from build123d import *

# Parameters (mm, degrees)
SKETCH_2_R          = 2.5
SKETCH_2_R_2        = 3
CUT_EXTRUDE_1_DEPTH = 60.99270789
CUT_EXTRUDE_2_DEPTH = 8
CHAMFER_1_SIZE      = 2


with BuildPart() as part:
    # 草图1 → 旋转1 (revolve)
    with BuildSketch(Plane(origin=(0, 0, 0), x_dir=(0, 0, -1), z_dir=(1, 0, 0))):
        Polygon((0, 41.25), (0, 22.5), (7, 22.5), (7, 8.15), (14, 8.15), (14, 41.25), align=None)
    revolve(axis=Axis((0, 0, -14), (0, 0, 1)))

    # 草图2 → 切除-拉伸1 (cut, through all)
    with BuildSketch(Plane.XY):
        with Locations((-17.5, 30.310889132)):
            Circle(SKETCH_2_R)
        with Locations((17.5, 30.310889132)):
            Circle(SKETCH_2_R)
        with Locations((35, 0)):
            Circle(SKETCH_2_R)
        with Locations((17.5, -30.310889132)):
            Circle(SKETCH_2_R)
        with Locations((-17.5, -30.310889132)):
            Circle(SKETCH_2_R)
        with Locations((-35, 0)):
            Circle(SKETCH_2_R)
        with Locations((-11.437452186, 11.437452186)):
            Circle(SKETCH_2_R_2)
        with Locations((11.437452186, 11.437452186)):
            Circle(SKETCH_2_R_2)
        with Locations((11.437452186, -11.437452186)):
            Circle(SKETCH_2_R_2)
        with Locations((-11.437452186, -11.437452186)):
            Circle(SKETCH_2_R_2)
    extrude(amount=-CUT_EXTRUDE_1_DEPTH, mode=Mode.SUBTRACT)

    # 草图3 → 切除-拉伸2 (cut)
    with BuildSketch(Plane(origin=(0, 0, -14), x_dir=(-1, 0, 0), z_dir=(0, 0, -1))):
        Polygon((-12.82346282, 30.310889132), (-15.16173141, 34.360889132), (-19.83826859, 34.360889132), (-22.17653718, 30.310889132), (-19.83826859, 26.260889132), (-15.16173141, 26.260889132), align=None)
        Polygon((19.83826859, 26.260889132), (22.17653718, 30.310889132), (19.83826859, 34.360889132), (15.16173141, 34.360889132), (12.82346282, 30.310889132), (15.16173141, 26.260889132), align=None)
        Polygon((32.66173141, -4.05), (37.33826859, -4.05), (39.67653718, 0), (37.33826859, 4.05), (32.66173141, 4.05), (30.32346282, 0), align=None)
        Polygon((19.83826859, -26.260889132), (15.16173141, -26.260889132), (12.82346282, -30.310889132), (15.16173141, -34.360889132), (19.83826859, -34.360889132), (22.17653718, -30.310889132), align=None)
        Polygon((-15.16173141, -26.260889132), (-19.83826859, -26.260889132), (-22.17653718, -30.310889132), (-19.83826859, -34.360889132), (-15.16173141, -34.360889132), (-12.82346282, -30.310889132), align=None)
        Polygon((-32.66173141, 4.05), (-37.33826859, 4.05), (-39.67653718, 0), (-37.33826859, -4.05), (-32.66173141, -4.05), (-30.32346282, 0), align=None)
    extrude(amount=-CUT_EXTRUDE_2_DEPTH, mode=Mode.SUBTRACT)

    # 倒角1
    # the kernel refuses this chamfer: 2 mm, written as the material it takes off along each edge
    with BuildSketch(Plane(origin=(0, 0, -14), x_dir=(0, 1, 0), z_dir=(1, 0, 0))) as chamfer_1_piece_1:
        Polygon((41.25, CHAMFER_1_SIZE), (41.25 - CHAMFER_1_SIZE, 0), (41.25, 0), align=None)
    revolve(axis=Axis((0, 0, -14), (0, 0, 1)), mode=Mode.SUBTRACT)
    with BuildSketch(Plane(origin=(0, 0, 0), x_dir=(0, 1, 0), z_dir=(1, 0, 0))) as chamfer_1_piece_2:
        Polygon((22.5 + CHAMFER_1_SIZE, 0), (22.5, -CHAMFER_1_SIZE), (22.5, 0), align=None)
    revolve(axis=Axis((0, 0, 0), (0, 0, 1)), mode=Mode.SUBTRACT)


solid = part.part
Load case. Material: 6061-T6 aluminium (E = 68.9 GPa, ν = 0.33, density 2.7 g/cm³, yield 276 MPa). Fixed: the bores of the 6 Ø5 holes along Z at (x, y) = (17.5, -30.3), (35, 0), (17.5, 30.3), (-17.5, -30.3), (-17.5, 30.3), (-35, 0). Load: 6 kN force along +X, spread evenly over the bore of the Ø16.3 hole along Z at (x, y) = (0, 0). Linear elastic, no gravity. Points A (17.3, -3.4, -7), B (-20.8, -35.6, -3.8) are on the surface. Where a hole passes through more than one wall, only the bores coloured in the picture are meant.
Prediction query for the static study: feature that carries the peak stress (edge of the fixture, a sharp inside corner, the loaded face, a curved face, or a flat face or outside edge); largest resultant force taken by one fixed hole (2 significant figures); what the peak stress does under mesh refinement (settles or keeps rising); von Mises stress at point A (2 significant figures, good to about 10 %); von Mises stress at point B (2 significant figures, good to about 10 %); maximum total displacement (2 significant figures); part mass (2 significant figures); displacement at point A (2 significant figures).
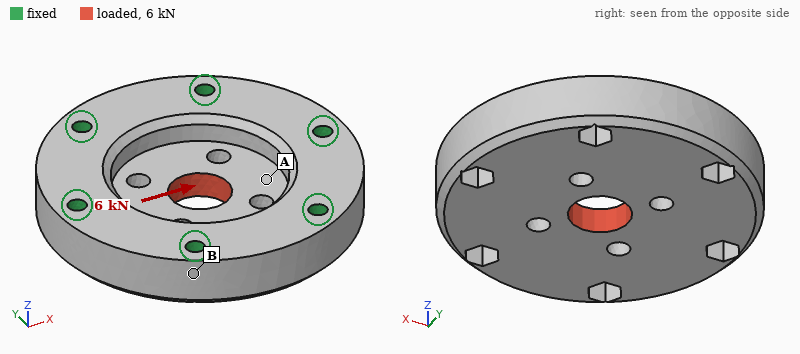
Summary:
edge of the fixture
1.3 kN
keeps rising
19 MPa
5.2 MPa
8.9 µm
150 g
5.8 µm
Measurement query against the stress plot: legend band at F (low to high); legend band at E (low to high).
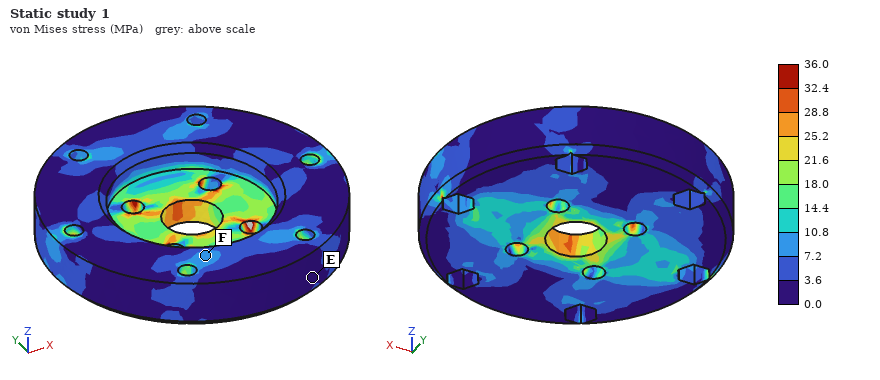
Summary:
7.2 to 10.8 MPa
0.0 to 3.6 MPa
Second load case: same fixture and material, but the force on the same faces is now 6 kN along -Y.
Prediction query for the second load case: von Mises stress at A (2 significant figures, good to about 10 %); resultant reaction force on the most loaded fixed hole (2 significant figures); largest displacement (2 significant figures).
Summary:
12 MPa
1.2 kN
9.0 µm
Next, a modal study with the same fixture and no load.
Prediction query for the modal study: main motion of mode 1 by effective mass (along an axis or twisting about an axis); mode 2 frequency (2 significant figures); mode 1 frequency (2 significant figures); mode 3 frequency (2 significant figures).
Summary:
along Z
21 kHz
16 kHz
21 kHz
